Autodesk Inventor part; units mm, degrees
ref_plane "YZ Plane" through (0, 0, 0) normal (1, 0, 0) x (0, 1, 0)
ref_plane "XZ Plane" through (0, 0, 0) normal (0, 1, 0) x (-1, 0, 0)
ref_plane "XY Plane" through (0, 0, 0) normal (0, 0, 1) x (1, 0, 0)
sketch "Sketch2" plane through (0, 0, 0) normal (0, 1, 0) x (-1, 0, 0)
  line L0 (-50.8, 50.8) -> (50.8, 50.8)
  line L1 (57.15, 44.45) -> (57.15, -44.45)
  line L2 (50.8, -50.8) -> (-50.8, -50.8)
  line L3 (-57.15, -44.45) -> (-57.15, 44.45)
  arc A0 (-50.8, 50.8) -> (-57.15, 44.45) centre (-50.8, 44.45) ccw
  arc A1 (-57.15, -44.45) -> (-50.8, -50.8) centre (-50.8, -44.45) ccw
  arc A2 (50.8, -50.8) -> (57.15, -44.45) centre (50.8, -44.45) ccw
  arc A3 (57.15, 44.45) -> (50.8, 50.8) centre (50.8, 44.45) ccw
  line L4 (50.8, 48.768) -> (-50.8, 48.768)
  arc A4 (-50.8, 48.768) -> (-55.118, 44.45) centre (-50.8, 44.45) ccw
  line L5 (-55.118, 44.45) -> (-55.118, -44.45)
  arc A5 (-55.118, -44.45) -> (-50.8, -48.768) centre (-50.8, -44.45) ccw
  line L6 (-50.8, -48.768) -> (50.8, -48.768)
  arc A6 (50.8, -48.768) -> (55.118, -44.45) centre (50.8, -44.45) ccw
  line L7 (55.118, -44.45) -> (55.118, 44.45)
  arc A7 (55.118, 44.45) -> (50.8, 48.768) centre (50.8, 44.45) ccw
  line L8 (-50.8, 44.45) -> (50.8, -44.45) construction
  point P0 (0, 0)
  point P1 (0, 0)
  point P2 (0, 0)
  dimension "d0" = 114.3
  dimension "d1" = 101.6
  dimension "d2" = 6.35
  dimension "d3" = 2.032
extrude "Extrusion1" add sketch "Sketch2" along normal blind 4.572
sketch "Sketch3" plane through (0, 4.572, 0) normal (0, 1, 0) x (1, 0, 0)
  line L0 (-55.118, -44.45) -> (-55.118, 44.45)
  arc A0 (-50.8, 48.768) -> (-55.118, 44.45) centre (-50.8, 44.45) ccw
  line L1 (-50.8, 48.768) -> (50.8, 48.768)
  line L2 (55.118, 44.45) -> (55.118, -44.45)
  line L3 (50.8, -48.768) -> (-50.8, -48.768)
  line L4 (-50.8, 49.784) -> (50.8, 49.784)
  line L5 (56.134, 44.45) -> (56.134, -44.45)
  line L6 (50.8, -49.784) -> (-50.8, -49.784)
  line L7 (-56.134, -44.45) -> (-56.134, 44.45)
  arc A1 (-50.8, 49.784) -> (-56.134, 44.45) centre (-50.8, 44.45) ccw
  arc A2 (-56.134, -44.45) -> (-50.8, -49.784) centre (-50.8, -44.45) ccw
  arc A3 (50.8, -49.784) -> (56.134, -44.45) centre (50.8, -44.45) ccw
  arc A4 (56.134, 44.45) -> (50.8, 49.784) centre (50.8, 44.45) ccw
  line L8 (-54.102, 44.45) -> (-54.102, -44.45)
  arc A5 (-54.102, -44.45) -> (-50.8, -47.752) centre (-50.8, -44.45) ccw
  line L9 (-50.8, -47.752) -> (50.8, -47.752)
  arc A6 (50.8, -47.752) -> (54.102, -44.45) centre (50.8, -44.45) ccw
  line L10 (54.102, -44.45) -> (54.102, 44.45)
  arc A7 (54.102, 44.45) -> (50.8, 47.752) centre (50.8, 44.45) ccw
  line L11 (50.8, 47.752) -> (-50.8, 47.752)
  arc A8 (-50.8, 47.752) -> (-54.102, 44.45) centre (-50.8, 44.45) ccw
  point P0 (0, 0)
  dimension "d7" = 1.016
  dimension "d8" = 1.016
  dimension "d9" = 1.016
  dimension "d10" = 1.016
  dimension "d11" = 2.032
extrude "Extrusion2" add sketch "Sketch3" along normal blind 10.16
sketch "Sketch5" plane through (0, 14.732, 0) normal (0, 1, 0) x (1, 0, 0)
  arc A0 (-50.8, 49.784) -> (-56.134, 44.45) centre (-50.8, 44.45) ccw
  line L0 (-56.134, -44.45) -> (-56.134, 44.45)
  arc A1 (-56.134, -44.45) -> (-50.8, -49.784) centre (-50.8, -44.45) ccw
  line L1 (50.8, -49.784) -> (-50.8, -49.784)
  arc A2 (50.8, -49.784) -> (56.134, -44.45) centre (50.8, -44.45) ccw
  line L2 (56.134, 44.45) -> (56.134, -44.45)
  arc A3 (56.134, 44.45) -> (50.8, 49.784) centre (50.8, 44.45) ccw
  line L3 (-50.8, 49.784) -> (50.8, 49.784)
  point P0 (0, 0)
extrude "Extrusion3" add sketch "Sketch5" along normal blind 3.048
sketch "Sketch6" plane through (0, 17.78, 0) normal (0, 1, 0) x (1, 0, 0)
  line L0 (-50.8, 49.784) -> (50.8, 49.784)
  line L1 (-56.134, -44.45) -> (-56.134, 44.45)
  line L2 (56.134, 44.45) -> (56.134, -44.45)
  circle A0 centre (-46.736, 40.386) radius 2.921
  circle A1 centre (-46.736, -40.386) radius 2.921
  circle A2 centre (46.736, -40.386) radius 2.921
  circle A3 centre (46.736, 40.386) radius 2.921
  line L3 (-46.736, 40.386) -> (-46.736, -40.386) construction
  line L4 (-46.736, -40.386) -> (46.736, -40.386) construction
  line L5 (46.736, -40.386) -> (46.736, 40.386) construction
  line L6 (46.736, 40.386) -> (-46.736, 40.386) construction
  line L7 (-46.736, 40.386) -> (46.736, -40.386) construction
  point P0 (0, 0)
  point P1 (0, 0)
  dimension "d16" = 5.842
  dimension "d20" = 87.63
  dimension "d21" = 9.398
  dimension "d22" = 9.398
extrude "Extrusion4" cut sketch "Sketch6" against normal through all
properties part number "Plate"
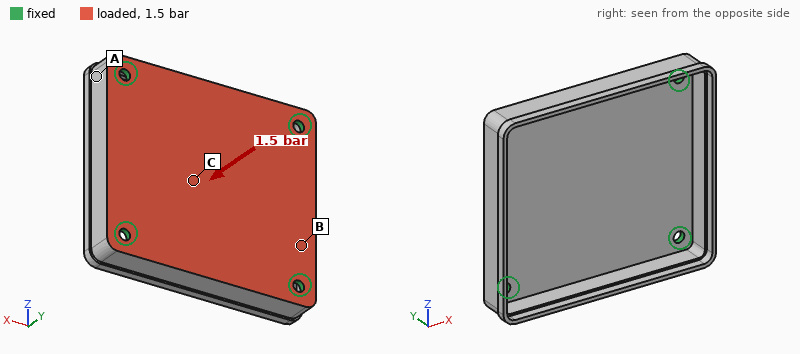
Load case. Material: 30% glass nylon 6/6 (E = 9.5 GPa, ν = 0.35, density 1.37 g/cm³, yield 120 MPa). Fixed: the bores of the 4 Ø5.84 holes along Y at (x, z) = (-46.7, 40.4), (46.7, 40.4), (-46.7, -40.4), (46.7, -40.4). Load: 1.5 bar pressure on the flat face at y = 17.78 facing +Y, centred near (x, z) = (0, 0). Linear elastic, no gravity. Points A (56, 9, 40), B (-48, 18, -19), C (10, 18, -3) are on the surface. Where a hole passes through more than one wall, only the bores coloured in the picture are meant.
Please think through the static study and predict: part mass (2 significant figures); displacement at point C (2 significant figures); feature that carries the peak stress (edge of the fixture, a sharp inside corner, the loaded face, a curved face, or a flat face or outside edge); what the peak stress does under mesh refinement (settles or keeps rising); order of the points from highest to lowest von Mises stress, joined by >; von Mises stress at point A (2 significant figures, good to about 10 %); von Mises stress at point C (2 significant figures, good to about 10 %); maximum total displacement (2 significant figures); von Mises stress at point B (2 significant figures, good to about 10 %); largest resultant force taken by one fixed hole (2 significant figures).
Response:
63 g
1.7 mm
edge of the fixture
keeps rising
C > B > A
11 MPa
36 MPa
1.7 mm
23 MPa
430 N
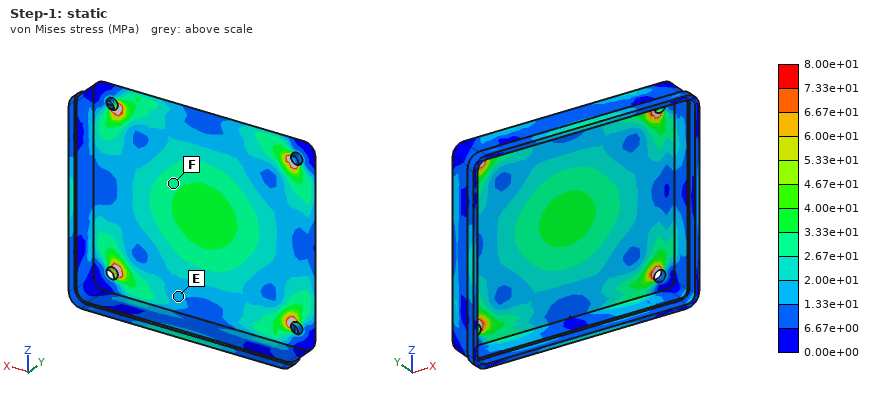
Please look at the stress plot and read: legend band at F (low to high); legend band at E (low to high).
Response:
2.67e+01 to 3.33e+01 MPa
1.33e+01 to 2.00e+01 MPa
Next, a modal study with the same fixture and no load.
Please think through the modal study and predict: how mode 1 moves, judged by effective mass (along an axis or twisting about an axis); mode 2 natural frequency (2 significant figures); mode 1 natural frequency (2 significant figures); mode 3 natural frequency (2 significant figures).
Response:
along Y
1900 Hz
900 Hz
1900 Hz
